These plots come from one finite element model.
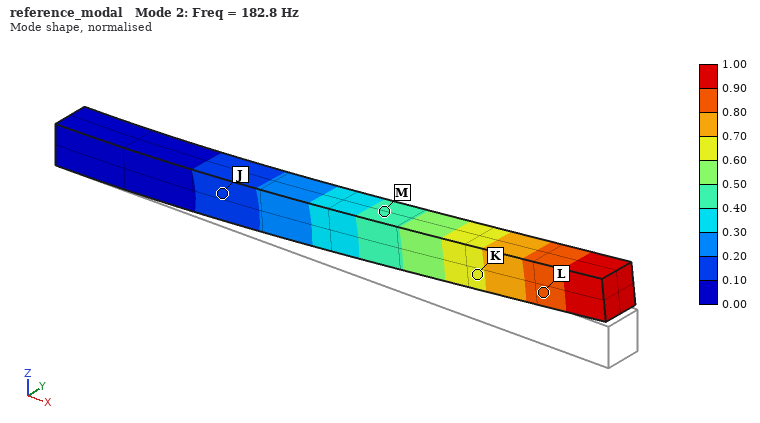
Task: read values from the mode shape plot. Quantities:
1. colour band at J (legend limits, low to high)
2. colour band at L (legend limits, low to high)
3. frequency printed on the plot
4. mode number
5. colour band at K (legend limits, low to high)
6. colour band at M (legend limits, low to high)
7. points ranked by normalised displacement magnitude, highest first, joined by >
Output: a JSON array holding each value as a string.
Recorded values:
["0.10 to 0.20", "0.80 to 0.90", "182.8 Hz", "2", "0.60 to 0.70", "0.40 to 0.50", "L > K > M > J"]
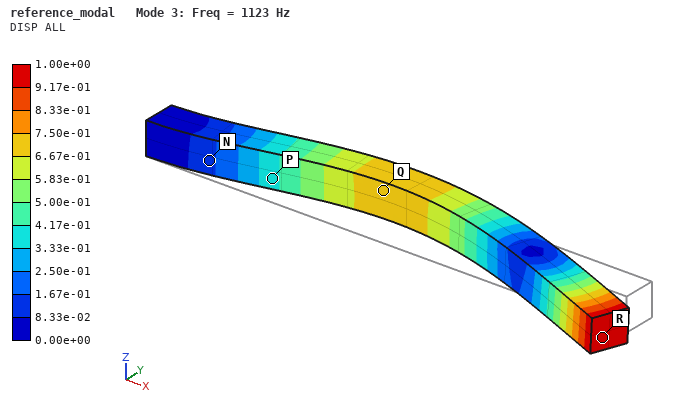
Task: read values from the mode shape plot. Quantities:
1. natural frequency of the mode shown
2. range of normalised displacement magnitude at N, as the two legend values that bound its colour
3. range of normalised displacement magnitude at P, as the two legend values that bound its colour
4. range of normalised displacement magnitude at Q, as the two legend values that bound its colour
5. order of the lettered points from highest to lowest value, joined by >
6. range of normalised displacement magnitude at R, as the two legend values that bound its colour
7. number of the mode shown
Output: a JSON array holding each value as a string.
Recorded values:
["1123 Hz", "8.33e-02 to 1.67e-01", "3.33e-01 to 4.17e-01", "6.67e-01 to 7.50e-01", "R > Q > P > N", "9.17e-01 to 1.00e+00", "3"]
